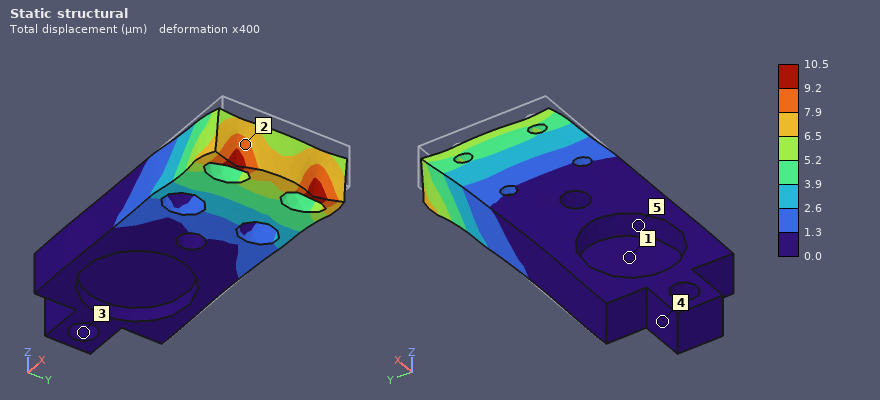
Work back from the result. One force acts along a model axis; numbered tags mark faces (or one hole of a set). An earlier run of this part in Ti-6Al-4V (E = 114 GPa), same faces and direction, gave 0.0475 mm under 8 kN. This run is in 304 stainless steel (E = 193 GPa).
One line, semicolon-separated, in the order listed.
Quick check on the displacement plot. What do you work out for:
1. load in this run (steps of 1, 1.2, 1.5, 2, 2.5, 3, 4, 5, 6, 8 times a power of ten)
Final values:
3 kN
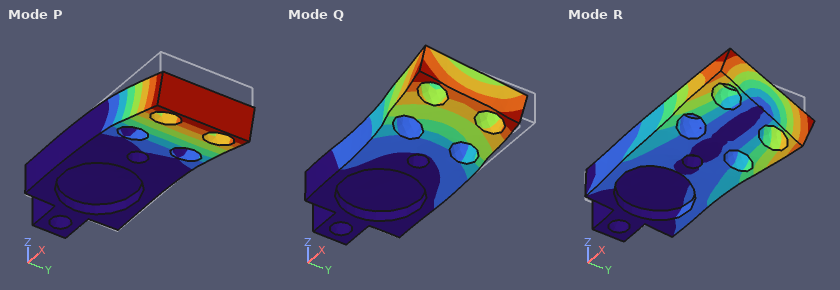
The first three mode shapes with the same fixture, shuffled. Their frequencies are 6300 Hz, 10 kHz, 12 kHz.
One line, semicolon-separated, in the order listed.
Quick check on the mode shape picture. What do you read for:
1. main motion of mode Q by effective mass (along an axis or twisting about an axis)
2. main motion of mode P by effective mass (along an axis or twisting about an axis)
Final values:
along Y; along Z
